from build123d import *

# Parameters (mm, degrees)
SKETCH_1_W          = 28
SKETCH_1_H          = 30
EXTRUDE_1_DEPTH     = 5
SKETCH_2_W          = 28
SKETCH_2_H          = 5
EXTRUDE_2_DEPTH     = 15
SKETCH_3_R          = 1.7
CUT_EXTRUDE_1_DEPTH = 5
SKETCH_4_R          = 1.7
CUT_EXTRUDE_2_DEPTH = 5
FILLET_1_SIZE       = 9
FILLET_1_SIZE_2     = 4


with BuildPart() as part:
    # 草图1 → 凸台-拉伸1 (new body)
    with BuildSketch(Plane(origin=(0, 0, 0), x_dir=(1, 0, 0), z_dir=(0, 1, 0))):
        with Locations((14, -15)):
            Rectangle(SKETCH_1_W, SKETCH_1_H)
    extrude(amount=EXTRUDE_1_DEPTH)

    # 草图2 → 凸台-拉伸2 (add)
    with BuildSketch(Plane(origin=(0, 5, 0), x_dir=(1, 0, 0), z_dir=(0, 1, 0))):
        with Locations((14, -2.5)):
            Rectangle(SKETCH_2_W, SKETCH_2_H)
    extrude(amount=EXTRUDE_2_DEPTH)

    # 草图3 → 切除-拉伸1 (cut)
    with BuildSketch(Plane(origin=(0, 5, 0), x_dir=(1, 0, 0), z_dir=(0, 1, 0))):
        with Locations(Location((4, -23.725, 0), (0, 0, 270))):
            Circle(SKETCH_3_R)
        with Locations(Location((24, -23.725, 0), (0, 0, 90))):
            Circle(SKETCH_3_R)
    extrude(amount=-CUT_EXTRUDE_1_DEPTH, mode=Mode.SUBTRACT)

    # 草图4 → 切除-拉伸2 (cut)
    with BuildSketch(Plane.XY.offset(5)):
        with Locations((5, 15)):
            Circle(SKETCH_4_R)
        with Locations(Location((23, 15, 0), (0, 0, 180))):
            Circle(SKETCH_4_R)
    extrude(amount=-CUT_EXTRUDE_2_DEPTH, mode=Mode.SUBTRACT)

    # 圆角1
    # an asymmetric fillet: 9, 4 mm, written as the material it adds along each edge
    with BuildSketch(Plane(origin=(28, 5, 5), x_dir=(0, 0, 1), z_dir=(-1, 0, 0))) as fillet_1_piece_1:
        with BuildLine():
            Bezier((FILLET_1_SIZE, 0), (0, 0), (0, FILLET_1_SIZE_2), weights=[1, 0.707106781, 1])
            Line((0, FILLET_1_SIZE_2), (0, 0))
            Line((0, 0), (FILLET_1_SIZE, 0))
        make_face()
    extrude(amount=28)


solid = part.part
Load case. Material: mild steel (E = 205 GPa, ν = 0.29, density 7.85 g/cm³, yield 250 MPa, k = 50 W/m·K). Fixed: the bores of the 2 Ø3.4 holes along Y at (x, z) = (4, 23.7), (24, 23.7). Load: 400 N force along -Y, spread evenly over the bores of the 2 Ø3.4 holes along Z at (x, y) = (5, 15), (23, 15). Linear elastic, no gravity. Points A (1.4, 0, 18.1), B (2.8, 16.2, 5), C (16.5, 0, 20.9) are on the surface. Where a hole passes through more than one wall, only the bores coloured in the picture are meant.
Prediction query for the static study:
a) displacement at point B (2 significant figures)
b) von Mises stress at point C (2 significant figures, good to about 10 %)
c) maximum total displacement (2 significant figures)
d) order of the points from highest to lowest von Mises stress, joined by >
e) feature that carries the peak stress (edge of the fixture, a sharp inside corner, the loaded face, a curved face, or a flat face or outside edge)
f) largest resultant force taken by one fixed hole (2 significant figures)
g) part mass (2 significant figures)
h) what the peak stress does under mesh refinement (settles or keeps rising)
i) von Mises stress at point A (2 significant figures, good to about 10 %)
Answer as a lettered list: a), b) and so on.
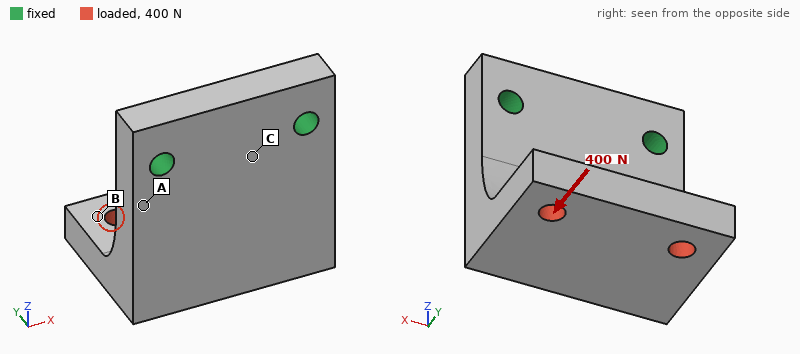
a) 28 µm
b) 36 MPa
c) 37 µm
d) A > C > B
e) edge of the fixture
f) 200 N
g) 50 g
h) keeps rising
i) 61 MPa
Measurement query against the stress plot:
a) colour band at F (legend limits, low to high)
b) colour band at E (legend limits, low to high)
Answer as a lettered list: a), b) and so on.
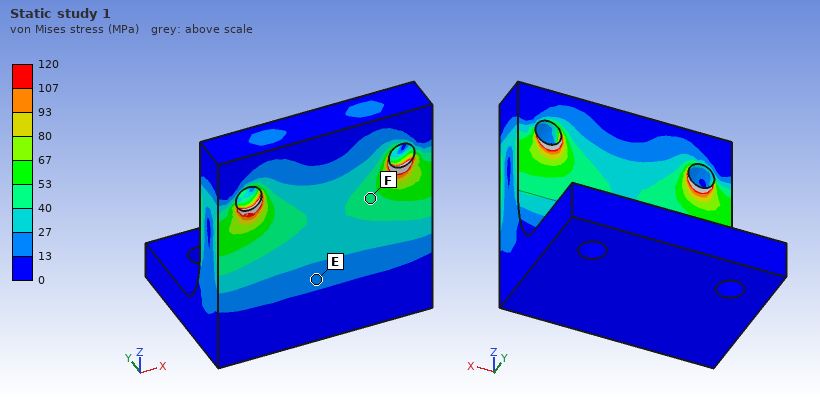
a) 40 to 53 MPa
b) 13 to 27 MPa
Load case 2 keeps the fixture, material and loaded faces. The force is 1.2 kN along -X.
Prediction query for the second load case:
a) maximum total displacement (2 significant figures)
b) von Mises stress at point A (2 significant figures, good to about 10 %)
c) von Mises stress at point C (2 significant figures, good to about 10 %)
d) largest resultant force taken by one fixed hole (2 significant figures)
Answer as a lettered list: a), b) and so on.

a) 39 µm
b) 80 MPa
c) 25 MPa
d) 1.5 kN
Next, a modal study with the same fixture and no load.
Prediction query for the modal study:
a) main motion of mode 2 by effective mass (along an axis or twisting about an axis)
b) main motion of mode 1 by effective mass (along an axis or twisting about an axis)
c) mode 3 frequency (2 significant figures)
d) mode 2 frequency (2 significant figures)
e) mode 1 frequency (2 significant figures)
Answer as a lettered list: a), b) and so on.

a) along X
b) along Y
c) 14 kHz
d) 7800 Hz
e) 3600 Hz
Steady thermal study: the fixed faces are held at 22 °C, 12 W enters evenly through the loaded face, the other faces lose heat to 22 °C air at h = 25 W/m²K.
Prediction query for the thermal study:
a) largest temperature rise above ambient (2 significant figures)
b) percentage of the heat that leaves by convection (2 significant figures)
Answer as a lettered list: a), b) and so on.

a) 50 K
b) 15 %
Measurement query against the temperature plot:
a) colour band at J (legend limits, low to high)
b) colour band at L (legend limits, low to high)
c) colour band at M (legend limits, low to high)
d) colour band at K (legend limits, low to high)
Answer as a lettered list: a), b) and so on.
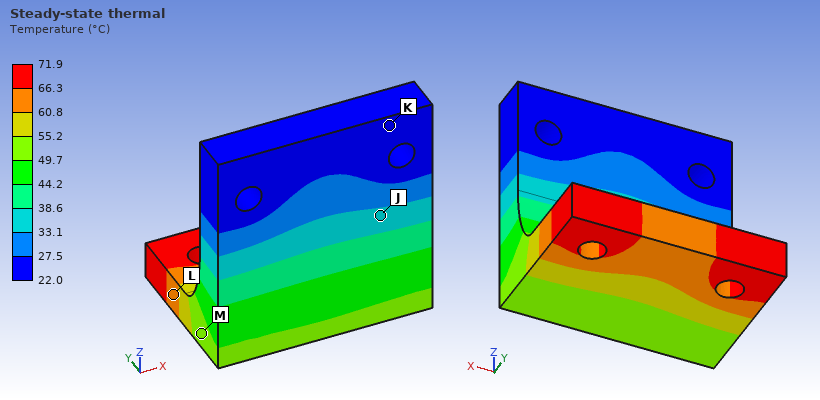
a) 33.1 to 38.6 °C
b) 60.8 to 66.3 °C
c) 49.7 to 55.2 °C
d) 22.0 to 27.5 °C
